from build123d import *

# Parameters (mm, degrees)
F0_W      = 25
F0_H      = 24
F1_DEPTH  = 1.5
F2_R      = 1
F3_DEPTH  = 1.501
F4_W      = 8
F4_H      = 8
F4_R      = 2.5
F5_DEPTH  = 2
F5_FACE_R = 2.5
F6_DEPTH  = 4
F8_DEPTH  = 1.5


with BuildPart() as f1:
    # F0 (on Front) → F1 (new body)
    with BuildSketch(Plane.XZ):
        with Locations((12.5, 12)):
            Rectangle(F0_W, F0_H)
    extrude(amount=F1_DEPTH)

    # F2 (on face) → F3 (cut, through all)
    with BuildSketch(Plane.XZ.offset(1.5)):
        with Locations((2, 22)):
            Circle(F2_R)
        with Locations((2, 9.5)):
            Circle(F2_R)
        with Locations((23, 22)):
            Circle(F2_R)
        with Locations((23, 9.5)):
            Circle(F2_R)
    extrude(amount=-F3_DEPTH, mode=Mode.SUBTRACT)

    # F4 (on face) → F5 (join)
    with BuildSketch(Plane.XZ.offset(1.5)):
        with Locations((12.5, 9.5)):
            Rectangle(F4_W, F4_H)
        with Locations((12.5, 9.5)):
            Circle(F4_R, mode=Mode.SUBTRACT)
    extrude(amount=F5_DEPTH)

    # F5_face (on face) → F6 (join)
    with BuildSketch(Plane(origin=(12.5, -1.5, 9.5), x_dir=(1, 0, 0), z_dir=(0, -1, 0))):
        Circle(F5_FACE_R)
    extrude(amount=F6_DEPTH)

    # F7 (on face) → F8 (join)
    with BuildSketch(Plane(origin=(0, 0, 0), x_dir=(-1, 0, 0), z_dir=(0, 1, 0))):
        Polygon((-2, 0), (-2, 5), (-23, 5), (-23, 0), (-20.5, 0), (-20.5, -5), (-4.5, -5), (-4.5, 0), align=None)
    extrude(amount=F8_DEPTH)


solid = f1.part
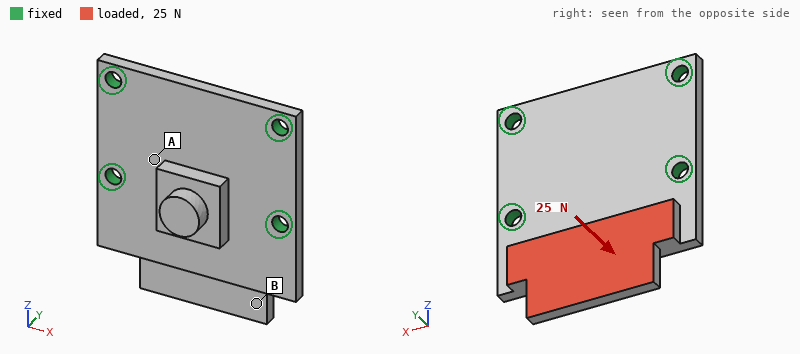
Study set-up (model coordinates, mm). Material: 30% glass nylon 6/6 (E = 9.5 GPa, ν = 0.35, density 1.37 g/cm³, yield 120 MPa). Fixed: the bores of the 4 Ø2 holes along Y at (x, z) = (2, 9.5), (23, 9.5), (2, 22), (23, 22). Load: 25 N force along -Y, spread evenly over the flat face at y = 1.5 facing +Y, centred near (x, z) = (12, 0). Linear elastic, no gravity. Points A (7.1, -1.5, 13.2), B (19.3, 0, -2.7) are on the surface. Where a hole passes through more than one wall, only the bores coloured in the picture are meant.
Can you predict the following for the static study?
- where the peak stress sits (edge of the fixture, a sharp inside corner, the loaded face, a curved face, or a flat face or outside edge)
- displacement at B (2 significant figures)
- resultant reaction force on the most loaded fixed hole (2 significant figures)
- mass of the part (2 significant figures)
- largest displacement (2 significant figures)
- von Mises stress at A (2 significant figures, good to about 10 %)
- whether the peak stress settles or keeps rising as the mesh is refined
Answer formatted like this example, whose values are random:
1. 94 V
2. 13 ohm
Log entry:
1. edge of the fixture
2. 0.12 mm
3. 17 N
4. 1.8 g
5. 0.16 mm
6. 6.0 MPa
7. keeps rising
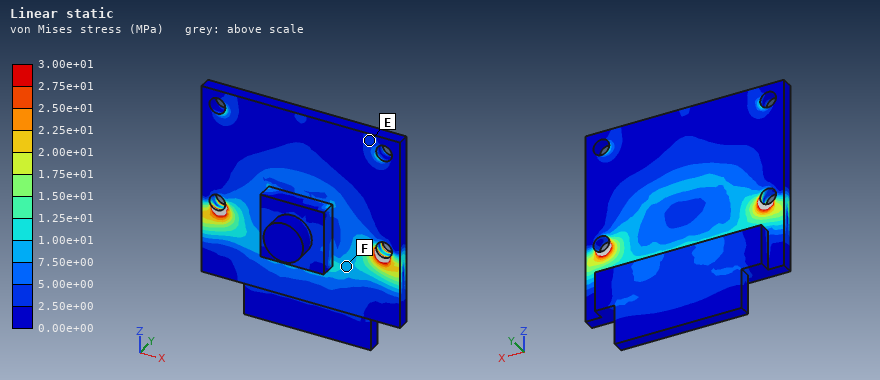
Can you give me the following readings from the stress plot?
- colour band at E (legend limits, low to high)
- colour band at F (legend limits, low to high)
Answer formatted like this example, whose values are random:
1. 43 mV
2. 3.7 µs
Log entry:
1. 2.50e+00 to 5.00e+00 MPa
2. 7.50e+00 to 1.00e+01 MPa
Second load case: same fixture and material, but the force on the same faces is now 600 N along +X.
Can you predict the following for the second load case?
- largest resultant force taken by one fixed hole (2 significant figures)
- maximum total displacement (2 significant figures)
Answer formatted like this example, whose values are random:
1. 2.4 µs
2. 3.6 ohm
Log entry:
1. 370 N
2. 0.16 mm
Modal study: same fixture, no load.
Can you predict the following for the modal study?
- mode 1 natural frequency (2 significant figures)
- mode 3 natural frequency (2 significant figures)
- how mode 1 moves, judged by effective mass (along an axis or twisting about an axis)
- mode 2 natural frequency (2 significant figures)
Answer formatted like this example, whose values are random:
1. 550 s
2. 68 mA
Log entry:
1. 3400 Hz
2. 9400 Hz
3. along Y
4. 9100 Hz
